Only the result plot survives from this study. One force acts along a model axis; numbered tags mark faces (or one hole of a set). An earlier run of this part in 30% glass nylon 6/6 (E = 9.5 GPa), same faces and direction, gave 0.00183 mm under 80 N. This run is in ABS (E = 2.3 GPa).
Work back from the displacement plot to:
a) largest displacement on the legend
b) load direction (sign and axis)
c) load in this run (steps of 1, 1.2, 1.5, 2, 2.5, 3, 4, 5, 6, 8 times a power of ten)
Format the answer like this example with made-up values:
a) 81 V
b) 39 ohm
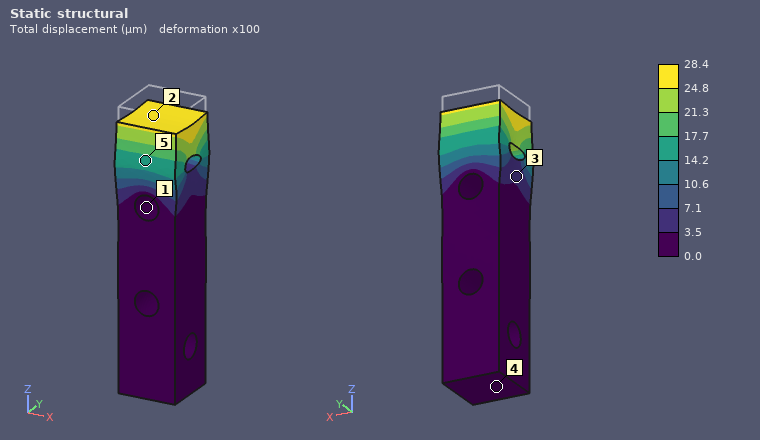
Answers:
a) 28.4 µm
b) -Z
c) 300 N
